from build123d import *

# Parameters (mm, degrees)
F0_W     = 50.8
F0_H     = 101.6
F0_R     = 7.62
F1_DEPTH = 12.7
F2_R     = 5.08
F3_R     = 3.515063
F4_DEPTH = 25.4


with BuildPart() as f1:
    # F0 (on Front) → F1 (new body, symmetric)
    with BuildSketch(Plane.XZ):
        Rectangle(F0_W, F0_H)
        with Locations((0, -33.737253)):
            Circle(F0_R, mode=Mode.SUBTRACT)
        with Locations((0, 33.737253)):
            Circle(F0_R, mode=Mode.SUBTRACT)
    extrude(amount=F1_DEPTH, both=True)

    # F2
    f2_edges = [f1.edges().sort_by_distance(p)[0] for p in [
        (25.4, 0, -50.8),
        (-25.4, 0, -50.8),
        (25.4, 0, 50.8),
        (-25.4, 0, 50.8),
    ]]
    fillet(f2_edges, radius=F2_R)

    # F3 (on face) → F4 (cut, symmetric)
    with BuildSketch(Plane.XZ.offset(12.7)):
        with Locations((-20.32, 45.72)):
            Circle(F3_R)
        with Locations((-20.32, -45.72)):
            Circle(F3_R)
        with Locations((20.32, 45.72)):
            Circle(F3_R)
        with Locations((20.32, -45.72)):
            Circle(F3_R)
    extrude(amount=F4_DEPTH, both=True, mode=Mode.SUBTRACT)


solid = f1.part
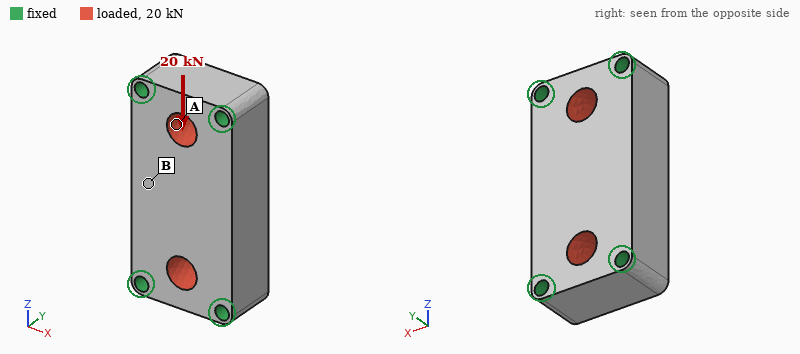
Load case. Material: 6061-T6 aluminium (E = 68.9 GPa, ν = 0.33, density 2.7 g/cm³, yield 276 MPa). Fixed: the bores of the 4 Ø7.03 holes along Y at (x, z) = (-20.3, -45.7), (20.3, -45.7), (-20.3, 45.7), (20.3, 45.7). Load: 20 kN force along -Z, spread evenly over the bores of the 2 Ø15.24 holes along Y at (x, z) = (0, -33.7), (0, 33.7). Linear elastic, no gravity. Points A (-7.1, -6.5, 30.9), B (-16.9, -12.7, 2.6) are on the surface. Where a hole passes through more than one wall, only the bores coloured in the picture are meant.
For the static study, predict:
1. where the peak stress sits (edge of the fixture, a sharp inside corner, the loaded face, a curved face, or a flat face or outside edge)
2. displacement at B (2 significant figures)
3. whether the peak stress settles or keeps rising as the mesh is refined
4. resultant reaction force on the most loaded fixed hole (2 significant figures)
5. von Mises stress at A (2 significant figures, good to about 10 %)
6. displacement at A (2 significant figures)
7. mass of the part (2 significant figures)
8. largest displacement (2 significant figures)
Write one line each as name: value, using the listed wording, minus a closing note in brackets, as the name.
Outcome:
where the peak stress sits: edge of the fixture
displacement at B: 2.9 µm
whether the peak stress settles or keeps rising as the mesh is refined: keeps rising
resultant reaction force on the most loaded fixed hole: 5.2 kN
von Mises stress at A: 14 MPa
displacement at A: 4.3 µm
mass of the part: 320 g
largest displacement: 6.8 µm
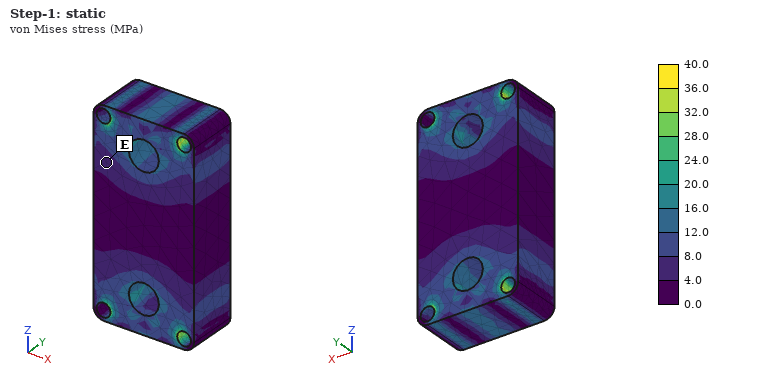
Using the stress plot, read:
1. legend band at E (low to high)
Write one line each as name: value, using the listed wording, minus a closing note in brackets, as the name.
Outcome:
legend band at E: 4.0 to 8.0 MPa
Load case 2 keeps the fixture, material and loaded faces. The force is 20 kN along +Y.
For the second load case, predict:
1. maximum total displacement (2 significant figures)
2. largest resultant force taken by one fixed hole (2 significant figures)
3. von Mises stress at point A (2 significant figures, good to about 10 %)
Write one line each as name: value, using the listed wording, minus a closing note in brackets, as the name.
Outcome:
maximum total displacement: 13 µm
largest resultant force taken by one fixed hole: 5.0 kN
von Mises stress at point A: 20 MPa
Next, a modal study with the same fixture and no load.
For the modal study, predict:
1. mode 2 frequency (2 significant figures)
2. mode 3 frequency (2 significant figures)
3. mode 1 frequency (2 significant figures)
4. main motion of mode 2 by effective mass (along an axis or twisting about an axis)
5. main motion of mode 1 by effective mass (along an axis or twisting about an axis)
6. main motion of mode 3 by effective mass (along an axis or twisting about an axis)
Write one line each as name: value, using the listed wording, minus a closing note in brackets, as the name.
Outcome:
mode 2 frequency: 12 kHz
mode 3 frequency: 14 kHz
mode 1 frequency: 10 kHz
main motion of mode 2 by effective mass: along X
main motion of mode 1 by effective mass: along Y
main motion of mode 3 by effective mass: twisting about Z
